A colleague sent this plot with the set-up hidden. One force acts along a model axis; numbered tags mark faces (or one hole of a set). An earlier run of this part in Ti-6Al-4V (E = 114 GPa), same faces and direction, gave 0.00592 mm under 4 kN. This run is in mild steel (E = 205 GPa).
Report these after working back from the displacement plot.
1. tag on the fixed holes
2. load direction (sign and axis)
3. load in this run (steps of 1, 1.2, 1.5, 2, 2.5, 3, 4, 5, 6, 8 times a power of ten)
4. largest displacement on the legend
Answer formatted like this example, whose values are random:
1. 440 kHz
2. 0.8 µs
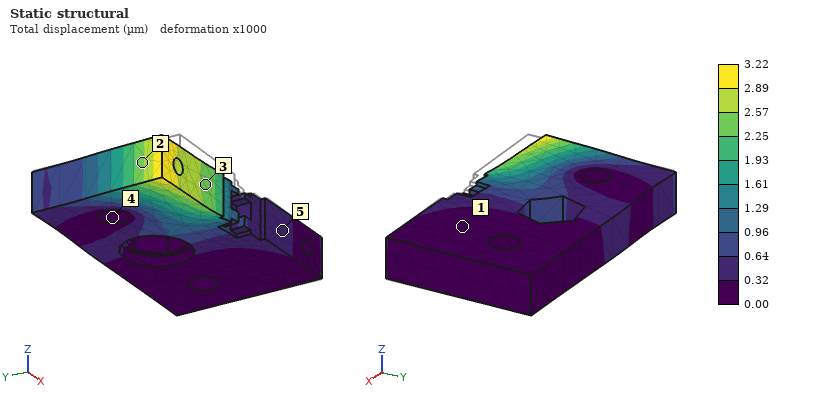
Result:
1. 4
2. +Y
3. 4 kN
4. 3.22 µm
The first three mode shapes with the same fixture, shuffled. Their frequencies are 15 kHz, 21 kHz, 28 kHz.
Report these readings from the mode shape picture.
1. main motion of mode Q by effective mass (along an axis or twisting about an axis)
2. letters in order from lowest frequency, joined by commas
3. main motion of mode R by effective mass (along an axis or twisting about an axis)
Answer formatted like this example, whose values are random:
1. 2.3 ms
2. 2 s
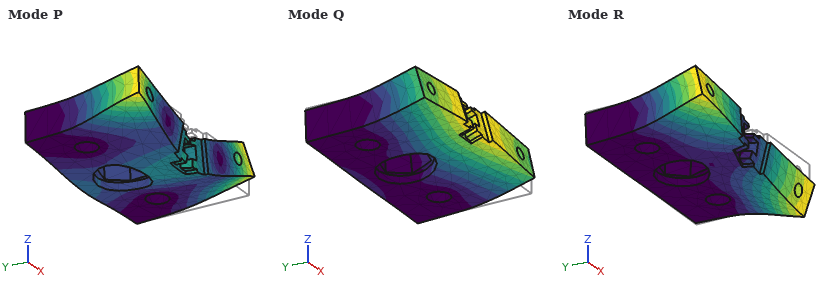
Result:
1. along Z
2. Q, R, P
3. twisting about Y
